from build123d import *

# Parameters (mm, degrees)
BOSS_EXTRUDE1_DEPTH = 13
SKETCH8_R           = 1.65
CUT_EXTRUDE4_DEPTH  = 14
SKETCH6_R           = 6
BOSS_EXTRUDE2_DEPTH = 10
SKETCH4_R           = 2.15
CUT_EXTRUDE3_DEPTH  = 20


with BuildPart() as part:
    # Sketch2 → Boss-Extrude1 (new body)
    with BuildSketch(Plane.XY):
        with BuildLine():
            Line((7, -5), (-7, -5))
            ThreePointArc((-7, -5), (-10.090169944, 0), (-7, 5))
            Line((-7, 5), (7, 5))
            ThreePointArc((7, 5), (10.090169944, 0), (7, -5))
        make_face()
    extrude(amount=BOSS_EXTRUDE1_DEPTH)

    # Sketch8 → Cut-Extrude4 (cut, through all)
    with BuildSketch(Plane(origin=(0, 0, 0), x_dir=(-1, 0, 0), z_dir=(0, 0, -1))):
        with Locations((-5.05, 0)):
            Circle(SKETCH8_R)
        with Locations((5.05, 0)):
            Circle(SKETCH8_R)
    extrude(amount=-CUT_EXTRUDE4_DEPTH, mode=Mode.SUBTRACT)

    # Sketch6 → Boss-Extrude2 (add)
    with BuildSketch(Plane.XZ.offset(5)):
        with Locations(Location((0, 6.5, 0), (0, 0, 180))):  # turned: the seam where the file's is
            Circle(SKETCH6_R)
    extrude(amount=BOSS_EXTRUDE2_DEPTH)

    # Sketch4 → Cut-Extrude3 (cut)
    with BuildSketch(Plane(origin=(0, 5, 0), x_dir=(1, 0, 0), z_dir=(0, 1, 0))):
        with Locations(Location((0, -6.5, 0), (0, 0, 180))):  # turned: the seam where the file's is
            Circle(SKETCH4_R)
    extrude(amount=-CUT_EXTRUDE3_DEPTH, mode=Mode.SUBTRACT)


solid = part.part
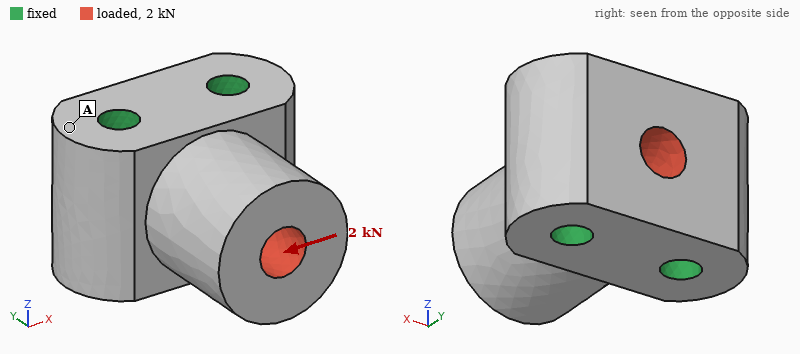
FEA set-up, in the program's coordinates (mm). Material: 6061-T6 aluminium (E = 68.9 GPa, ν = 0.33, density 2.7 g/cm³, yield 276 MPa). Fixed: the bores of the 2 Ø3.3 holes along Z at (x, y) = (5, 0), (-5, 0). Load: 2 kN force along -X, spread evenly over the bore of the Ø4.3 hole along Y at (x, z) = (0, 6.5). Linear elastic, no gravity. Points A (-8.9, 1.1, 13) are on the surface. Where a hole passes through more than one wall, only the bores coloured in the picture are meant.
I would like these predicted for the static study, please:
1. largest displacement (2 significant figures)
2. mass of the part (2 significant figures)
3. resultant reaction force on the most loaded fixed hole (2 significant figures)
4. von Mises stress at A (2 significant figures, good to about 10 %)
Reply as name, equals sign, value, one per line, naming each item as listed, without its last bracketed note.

largest displacement = 7.7 µm
mass of the part = 8.1 g
resultant reaction force on the most loaded fixed hole = 1.3 kN
von Mises stress at A = 4.1 MPa
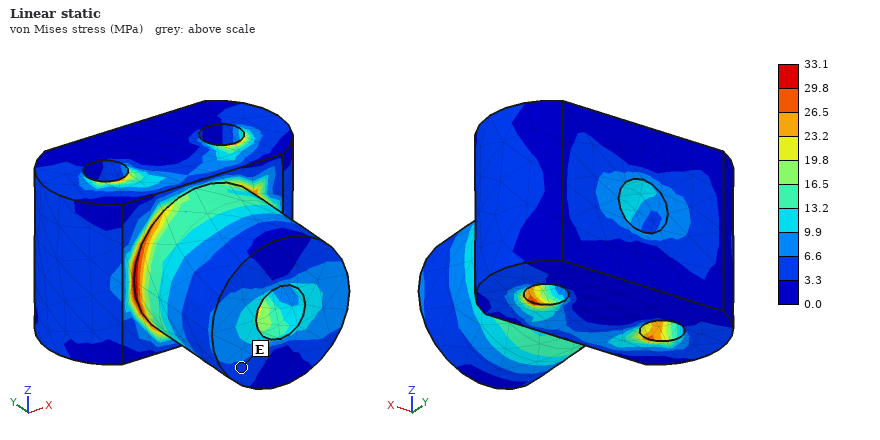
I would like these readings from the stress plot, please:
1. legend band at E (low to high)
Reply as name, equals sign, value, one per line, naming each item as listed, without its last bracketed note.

legend band at E = 3.3 to 6.6 MPa
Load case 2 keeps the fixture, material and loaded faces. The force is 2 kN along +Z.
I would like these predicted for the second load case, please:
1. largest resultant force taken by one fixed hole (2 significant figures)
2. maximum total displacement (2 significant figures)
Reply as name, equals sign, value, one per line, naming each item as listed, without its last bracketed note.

largest resultant force taken by one fixed hole = 1.0 kN
maximum total displacement = 9.9 µm
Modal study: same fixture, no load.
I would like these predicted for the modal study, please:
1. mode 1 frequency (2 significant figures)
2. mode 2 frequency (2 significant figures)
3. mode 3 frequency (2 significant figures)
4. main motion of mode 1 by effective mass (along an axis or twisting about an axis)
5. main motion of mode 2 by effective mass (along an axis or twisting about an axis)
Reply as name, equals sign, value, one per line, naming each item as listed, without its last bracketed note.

mode 1 frequency = 37 kHz
mode 2 frequency = 42 kHz
mode 3 frequency = 64 kHz
main motion of mode 1 by effective mass = along Z
main motion of mode 2 by effective mass = along X
